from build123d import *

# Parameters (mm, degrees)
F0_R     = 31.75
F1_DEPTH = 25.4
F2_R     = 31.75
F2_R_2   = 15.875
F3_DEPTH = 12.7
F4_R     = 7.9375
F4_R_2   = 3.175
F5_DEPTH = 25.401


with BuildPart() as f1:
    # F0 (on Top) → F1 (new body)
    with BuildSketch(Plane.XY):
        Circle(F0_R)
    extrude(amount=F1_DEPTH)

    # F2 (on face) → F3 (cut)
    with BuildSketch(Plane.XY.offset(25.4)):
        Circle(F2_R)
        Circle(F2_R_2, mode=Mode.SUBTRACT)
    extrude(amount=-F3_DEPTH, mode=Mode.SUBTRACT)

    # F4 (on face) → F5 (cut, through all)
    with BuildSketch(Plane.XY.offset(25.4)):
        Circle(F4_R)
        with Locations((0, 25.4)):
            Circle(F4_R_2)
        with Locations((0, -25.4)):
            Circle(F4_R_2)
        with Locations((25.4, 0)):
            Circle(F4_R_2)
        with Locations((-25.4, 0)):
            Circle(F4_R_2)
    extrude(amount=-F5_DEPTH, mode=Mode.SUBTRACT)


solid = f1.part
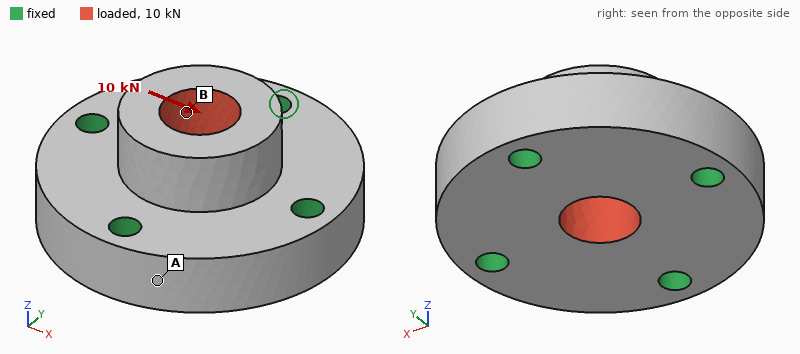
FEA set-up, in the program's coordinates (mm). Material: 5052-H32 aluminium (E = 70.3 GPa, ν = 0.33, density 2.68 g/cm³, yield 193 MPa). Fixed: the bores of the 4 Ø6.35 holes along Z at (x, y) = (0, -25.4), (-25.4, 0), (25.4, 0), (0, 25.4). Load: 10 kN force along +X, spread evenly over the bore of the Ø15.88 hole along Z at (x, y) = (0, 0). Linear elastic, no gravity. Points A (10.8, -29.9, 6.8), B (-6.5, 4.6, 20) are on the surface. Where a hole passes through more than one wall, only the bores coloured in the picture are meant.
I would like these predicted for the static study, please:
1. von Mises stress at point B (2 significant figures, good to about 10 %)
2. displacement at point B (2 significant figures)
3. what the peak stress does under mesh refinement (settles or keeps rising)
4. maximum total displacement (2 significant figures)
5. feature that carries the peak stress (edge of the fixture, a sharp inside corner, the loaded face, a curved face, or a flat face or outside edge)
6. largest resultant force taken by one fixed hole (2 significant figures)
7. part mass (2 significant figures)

15 MPa
8.3 µm
keeps rising
11 µm
edge of the fixture
3.4 kN
120 g
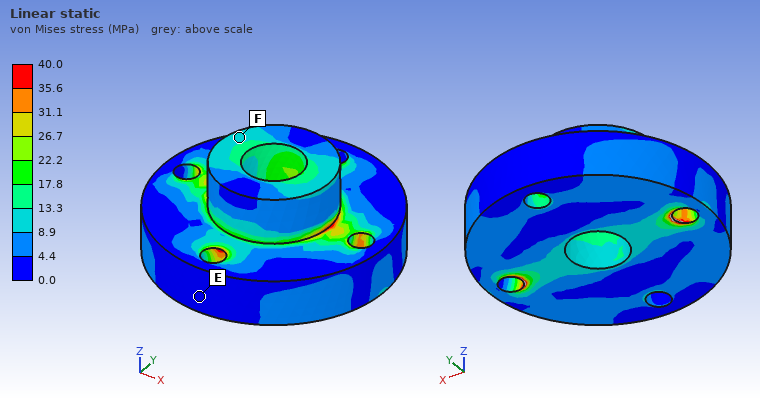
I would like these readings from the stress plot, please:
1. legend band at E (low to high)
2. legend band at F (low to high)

0.0 to 4.4 MPa
8.9 to 13.3 MPa
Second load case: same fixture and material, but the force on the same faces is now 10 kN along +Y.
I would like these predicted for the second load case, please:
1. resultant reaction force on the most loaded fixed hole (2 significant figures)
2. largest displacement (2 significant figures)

3.4 kN
11 µm
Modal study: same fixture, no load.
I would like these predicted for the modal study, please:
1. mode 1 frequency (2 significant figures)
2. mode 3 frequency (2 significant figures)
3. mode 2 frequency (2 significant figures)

25 kHz
26 kHz
26 kHz
